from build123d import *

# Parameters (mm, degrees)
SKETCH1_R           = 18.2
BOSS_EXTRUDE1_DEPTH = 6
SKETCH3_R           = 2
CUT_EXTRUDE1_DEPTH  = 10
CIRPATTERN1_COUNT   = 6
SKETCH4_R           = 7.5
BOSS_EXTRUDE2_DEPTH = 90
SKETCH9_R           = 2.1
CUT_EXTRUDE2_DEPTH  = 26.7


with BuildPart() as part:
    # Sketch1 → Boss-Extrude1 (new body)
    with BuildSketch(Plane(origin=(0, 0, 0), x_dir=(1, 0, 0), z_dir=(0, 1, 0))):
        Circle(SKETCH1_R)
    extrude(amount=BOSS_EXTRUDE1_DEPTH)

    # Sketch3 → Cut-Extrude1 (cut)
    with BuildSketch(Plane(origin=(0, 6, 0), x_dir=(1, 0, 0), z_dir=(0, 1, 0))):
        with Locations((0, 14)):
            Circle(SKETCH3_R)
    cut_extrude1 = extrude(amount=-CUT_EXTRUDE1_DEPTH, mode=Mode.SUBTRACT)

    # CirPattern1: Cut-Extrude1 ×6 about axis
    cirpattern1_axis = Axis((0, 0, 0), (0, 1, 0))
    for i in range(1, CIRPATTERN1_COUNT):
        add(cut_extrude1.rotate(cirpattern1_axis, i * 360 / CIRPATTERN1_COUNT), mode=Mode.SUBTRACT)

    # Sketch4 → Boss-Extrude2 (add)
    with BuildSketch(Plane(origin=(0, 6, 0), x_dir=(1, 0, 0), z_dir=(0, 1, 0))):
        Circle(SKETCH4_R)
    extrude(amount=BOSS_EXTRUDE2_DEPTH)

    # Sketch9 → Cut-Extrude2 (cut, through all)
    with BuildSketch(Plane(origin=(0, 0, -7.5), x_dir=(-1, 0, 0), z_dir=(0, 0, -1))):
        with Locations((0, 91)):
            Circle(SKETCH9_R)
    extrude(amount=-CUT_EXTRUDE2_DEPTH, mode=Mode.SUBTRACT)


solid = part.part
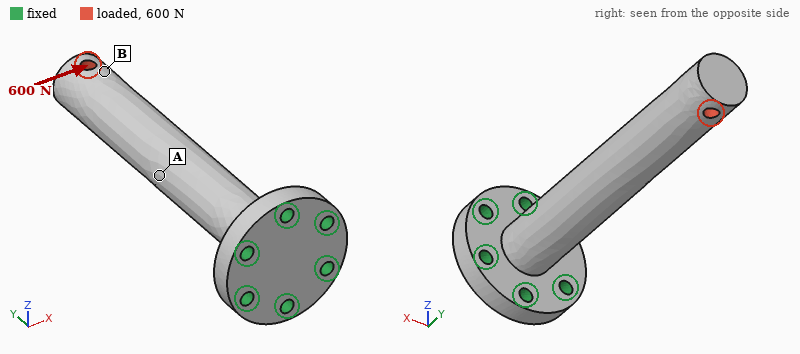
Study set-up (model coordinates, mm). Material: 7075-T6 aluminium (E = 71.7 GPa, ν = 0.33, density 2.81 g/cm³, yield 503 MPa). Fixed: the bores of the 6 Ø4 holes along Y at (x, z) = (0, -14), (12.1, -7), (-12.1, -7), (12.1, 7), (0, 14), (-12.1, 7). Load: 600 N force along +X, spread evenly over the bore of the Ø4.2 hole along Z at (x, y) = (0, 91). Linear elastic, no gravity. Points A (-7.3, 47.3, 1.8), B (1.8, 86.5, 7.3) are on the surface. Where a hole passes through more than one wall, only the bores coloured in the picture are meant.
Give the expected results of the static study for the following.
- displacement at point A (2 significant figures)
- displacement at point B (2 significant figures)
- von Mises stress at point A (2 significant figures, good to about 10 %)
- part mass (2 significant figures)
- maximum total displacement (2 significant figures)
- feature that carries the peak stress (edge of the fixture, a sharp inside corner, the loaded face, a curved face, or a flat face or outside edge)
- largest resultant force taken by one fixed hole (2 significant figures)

0.28 mm
0.77 mm
77 MPa
60 g
0.90 mm
a curved face
1.3 kN
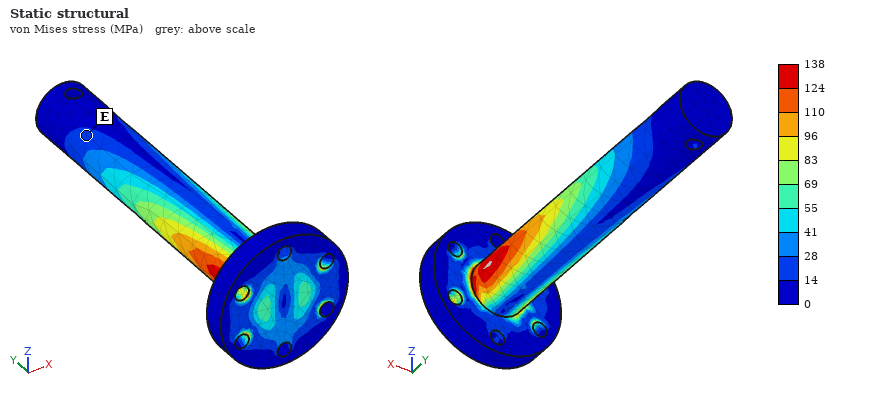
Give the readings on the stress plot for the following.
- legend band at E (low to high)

14 to 28 MPa
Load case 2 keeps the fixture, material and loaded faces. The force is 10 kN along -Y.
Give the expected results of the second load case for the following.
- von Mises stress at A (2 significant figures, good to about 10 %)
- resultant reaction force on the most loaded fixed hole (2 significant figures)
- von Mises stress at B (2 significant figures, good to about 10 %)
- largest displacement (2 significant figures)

56 MPa
1.8 kN
68 MPa
90 µm
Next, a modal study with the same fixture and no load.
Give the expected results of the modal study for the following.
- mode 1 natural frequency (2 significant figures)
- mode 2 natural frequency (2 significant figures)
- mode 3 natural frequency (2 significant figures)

1200 Hz
1200 Hz
6900 Hz
